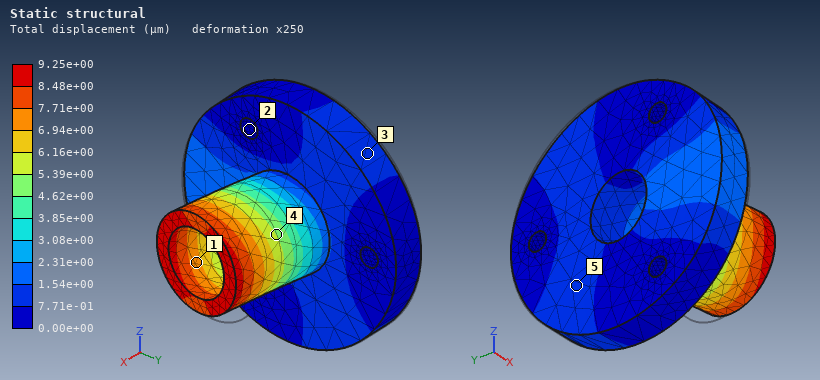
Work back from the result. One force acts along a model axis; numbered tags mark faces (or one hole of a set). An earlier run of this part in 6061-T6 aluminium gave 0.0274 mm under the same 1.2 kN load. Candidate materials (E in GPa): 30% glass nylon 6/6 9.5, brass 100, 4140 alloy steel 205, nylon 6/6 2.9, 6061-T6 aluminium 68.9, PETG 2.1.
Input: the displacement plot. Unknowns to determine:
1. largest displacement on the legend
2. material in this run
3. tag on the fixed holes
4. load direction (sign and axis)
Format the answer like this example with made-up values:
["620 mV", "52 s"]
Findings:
["9.25e+00 µm", "4140 alloy steel", "2", "-Y"]
